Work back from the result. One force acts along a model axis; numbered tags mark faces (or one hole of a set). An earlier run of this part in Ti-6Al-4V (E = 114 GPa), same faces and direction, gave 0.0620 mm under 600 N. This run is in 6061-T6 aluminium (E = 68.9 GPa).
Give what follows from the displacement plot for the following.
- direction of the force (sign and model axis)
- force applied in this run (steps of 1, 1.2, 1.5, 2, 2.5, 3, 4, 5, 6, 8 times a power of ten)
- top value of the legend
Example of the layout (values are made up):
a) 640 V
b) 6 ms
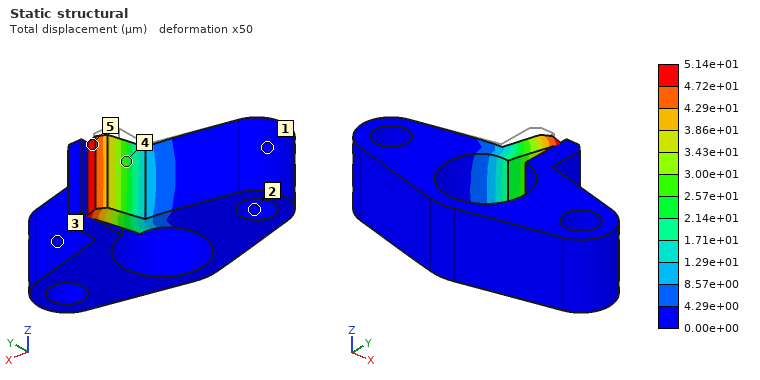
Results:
a) +X
b) 300 N
c) 5.14e+01 µm
